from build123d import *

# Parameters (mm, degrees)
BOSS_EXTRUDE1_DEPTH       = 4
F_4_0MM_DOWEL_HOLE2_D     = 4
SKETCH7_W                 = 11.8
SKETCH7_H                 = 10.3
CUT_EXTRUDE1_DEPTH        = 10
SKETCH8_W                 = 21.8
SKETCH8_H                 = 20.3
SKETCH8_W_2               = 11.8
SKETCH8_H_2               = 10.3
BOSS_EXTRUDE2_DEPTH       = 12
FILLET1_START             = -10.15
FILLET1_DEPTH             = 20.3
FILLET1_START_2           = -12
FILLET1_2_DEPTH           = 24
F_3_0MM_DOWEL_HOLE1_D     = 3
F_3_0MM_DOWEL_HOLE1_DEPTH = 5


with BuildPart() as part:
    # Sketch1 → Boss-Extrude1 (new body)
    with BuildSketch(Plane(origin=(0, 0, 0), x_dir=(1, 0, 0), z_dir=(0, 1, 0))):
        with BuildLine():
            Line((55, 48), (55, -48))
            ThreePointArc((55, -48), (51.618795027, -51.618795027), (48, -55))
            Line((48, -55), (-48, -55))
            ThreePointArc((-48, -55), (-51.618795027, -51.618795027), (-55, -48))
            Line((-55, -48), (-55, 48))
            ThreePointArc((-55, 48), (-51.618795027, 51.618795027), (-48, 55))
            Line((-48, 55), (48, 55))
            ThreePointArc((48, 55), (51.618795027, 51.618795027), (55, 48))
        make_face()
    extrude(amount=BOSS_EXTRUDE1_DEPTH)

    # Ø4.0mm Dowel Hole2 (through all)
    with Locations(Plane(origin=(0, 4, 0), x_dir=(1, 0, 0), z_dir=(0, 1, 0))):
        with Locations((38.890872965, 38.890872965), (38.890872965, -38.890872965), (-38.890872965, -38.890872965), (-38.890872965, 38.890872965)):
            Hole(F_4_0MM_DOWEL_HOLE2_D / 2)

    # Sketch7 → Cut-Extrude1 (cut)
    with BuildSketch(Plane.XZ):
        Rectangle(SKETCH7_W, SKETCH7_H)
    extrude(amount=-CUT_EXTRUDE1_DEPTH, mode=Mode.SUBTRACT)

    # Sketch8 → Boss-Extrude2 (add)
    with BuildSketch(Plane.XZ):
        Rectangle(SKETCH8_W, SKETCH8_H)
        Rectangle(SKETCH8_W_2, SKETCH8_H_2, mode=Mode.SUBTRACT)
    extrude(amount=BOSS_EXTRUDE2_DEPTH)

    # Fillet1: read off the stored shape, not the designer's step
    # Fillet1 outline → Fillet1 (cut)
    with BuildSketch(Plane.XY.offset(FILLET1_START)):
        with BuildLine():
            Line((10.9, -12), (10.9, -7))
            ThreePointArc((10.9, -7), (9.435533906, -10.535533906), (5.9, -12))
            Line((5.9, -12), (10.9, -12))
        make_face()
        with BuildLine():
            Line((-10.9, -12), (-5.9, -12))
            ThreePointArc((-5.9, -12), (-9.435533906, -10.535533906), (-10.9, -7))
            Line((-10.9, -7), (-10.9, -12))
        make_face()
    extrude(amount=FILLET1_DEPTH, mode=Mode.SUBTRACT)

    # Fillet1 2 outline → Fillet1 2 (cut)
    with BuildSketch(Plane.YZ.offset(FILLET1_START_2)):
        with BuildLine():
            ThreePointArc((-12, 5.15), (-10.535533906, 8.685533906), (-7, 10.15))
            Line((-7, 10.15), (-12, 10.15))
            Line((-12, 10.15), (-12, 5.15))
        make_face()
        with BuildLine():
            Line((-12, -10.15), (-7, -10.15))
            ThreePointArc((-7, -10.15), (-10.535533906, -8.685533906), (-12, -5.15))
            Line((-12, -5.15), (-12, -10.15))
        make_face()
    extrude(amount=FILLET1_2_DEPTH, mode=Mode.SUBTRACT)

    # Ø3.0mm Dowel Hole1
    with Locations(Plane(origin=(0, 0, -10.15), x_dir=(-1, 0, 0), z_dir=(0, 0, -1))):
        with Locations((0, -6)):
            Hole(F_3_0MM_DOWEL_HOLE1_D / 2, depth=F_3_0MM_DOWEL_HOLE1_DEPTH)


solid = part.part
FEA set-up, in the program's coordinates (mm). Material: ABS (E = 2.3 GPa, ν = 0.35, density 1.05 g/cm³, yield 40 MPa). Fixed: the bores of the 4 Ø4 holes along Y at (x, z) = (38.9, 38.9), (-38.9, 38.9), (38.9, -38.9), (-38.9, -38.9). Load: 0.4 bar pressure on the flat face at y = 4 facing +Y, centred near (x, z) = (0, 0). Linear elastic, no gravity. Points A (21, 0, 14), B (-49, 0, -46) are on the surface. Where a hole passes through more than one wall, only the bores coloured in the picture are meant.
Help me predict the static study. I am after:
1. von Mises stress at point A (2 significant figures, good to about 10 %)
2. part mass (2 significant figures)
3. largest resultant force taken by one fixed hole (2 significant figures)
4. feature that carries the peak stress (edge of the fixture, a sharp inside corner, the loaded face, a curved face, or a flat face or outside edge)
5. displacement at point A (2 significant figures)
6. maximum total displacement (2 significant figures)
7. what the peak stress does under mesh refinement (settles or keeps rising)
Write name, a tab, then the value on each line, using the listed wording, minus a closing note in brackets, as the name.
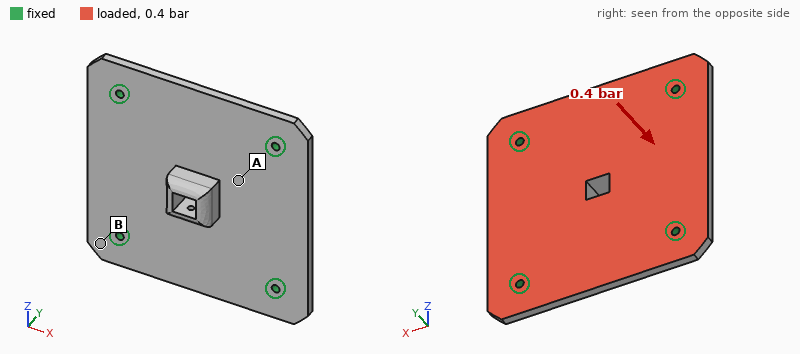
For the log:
von Mises stress at point A	3.5 MPa
part mass	53 g
largest resultant force taken by one fixed hole	120 N
feature that carries the peak stress	edge of the fixture
displacement at point A	0.52 mm
maximum total displacement	0.63 mm
what the peak stress does under mesh refinement	keeps rising
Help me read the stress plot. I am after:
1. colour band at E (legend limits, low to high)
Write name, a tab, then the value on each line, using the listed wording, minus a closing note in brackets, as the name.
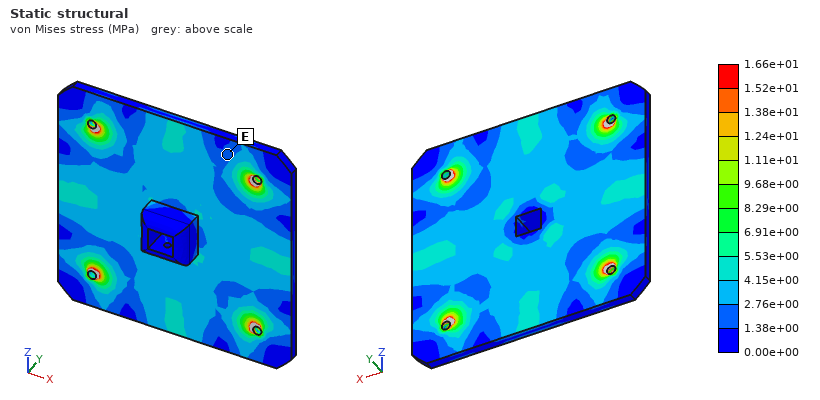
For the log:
colour band at E	1.38e+00 to 2.76e+00 MPa
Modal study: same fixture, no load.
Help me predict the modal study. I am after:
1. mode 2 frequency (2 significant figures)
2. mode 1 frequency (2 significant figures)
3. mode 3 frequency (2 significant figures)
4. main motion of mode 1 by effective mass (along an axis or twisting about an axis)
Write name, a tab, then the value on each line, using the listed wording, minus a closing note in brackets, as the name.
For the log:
mode 2 frequency	990 Hz
mode 1 frequency	640 Hz
mode 3 frequency	990 Hz
main motion of mode 1 by effective mass	along Y
